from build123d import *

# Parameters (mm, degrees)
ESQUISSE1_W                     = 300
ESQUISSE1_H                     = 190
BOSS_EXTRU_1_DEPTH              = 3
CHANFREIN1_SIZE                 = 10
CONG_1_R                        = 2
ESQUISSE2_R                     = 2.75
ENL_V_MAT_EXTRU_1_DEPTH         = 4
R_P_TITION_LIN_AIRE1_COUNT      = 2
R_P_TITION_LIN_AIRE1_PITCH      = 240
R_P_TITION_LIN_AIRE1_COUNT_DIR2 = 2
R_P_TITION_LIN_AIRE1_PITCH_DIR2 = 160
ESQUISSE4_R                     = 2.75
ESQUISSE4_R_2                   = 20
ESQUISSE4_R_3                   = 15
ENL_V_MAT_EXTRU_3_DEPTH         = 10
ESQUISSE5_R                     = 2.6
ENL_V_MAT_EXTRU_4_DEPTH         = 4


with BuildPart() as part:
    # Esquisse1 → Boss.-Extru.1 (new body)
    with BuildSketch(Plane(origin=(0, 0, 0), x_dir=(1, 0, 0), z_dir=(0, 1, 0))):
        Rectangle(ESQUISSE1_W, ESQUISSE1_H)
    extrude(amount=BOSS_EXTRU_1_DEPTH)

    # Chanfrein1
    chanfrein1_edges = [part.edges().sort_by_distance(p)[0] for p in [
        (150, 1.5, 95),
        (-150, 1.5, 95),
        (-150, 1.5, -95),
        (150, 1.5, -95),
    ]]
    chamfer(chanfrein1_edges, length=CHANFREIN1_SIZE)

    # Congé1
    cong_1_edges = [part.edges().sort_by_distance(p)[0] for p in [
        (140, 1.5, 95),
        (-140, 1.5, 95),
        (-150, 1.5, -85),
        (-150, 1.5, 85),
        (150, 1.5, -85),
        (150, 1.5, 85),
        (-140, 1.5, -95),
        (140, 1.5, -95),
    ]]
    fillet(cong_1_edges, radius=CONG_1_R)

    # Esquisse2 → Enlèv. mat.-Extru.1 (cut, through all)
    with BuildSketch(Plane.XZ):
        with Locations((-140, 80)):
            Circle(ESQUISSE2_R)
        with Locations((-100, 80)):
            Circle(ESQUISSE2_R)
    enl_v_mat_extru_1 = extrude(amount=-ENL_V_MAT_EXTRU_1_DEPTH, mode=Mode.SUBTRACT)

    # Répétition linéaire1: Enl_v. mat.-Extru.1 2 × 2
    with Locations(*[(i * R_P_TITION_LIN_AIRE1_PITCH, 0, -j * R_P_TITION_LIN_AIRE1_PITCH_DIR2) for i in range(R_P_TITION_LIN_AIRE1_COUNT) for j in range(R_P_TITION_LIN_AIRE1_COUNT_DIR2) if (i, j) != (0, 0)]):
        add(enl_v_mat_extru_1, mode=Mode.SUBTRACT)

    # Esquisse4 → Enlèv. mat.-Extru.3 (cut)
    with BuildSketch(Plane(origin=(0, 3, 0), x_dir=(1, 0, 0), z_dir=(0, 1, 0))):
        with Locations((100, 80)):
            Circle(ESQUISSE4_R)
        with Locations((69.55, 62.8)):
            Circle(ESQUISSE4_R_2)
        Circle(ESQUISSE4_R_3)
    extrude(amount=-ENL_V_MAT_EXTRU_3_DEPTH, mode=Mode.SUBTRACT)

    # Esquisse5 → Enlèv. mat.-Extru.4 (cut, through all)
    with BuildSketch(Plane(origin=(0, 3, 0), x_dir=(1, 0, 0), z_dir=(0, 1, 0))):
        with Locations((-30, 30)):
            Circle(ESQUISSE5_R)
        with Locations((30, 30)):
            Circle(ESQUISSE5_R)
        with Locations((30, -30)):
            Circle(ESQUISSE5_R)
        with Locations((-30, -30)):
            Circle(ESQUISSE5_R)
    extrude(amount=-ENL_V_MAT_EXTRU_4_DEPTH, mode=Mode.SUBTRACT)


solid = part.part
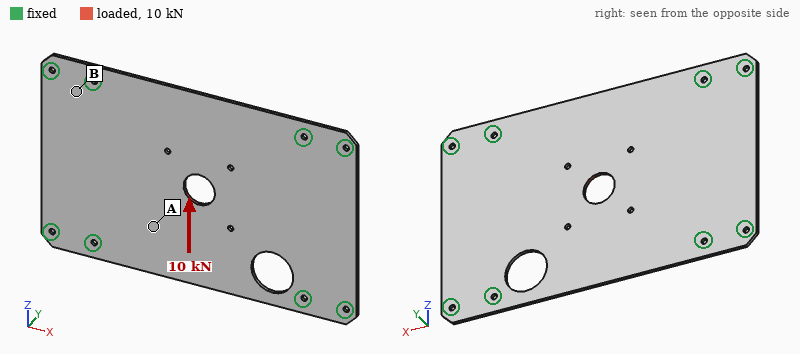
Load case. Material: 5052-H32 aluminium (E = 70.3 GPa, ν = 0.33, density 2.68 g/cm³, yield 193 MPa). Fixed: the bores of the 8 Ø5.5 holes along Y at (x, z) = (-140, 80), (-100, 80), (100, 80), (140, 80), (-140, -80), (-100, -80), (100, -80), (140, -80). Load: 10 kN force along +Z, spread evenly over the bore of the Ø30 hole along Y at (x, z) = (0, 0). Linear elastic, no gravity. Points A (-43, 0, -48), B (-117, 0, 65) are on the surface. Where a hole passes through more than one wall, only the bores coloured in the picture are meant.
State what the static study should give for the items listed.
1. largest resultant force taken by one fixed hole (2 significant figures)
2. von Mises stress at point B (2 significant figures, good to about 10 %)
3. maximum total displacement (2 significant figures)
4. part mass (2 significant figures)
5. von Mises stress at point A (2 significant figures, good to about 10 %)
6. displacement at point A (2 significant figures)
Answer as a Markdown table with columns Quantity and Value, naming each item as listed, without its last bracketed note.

| Quantity | Value |
|---|---|
| largest resultant force taken by one fixed hole | 2.7 kN |
| von Mises stress at point B | 8.8 MPa |
| maximum total displacement | 60 µm |
| part mass | 440 g |
| von Mises stress at point A | 18 MPa |
| displacement at point A | 33 µm |
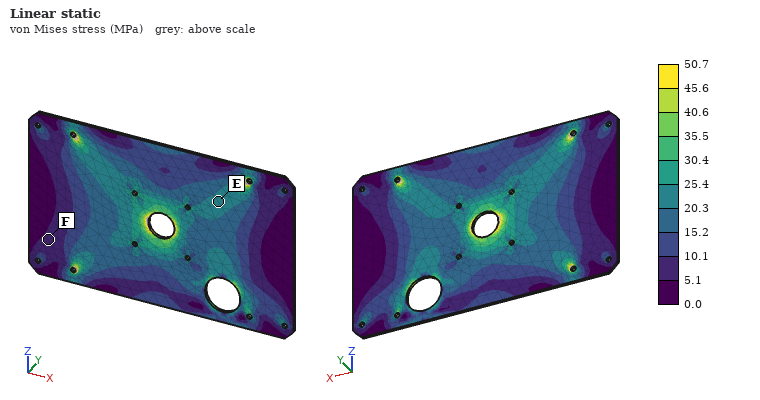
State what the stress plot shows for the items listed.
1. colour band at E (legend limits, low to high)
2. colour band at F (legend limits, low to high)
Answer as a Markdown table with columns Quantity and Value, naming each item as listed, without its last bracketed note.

| Quantity | Value |
|---|---|
| colour band at E | 20.3 to 25.4 MPa |
| colour band at F | 5.1 to 10.1 MPa |
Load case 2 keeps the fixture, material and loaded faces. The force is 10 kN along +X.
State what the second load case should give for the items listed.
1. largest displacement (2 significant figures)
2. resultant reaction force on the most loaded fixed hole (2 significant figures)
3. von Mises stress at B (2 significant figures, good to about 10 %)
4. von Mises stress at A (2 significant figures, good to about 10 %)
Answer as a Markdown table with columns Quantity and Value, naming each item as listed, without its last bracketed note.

| Quantity | Value |
|---|---|
| largest displacement | 41 µm |
| resultant reaction force on the most loaded fixed hole | 2.1 kN |
| von Mises stress at B | 15 MPa |
| von Mises stress at A | 13 MPa |
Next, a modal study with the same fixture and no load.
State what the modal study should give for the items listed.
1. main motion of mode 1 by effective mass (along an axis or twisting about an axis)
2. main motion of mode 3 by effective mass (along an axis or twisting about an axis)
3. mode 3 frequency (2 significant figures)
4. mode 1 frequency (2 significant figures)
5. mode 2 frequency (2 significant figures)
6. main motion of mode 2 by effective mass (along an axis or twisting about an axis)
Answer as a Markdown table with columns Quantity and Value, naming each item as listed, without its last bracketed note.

| Quantity | Value |
|---|---|
| main motion of mode 1 by effective mass | along Y |
| main motion of mode 3 by effective mass | twisting about Z |
| mode 3 frequency | 610 Hz |
| mode 1 frequency | 300 Hz |
| mode 2 frequency | 460 Hz |
| main motion of mode 2 by effective mass | twisting about X |
